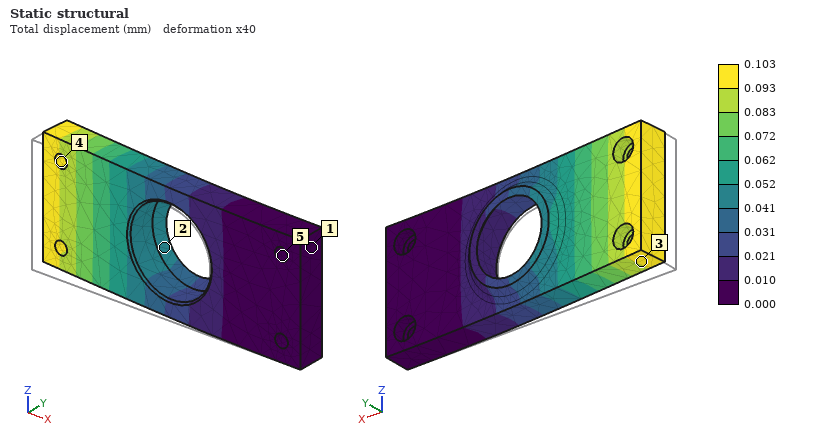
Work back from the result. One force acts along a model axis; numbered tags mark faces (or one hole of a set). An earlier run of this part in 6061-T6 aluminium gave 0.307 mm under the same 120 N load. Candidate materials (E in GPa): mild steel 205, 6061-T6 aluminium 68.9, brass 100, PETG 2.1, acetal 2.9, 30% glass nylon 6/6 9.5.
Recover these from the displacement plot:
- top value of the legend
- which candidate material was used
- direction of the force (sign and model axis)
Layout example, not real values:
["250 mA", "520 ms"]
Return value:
["0.103 mm", "mild steel", "+Y"]
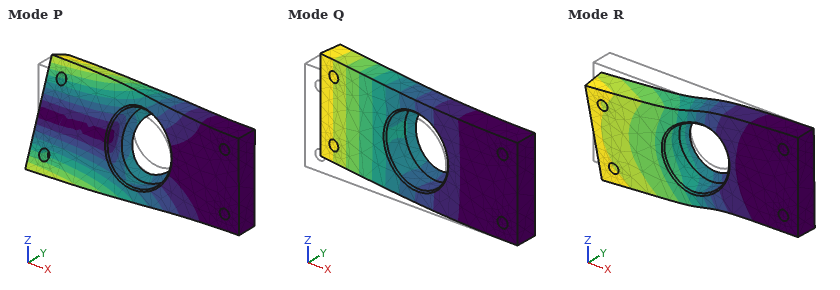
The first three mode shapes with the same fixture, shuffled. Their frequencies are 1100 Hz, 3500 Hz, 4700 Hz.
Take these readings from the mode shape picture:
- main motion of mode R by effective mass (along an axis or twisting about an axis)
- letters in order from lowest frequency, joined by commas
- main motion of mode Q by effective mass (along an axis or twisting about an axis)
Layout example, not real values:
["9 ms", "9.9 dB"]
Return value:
["along Z", "Q, R, P", "along Y"]
